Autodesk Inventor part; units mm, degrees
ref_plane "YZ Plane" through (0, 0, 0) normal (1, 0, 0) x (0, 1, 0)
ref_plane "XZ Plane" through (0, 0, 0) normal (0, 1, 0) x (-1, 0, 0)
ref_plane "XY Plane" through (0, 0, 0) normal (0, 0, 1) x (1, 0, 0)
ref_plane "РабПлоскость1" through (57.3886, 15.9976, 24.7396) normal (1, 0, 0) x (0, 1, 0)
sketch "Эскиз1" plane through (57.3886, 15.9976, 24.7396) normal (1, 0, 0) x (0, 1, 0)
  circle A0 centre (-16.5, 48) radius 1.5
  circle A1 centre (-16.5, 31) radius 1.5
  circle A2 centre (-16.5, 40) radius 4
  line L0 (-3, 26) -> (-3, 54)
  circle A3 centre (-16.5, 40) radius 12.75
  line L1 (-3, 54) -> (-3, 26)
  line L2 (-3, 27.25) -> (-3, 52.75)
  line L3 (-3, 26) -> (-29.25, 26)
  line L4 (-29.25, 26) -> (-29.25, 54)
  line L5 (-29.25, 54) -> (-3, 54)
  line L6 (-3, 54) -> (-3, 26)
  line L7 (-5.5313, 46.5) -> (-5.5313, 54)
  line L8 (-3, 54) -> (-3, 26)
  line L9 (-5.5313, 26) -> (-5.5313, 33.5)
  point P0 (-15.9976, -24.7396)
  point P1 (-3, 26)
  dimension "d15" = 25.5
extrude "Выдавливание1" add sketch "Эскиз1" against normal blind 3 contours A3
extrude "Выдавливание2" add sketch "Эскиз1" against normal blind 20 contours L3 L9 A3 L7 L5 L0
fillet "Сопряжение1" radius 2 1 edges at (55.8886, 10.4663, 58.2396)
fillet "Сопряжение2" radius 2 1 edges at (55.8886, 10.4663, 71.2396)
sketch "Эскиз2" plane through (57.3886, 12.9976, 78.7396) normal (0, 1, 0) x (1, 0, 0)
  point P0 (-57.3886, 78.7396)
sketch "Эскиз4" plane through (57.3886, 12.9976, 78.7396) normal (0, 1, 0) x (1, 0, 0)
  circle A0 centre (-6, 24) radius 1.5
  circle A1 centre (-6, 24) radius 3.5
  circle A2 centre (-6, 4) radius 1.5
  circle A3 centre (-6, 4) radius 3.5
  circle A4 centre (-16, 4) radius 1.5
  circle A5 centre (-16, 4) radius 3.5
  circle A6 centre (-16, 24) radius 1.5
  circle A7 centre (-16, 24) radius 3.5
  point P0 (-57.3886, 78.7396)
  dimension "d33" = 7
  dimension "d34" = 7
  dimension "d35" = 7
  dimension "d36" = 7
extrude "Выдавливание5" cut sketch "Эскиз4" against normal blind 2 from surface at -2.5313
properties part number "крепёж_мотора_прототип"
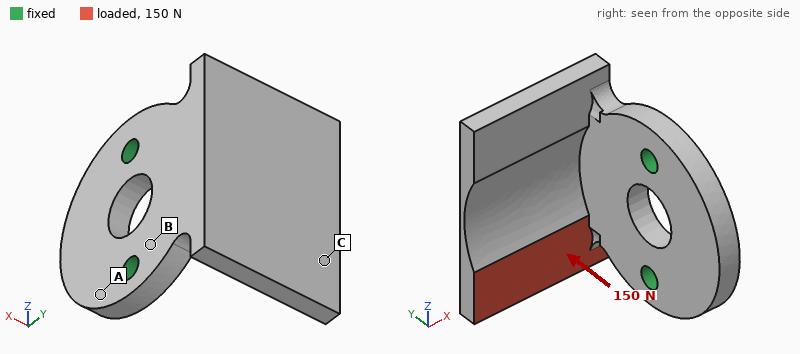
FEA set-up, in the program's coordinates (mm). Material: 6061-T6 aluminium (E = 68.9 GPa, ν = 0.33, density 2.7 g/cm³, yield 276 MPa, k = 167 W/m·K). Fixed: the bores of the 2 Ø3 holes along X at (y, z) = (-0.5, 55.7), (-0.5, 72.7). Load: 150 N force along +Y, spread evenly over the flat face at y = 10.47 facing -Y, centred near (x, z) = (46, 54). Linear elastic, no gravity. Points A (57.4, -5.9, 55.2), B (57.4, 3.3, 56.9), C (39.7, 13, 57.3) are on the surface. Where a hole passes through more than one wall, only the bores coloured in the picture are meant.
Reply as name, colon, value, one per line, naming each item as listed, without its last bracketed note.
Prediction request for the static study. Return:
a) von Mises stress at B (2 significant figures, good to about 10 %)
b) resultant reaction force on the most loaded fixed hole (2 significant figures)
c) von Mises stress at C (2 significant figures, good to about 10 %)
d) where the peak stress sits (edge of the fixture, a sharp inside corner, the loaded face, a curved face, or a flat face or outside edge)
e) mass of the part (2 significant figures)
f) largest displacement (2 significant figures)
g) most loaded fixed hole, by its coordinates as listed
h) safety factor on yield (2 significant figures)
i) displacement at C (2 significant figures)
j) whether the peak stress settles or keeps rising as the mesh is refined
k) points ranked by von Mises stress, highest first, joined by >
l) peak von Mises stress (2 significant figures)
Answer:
von Mises stress at B: 50 MPa
resultant reaction force on the most loaded fixed hole: 160 N
von Mises stress at C: 24 MPa
where the peak stress sits: a curved face
mass of the part: 6.7 g
largest displacement: 0.28 mm
most loaded fixed hole, by its coordinates as listed: (-0.5, 55.7)
safety factor on yield: 1.3
displacement at C: 0.21 mm
whether the peak stress settles or keeps rising as the mesh is refined: settles
points ranked by von Mises stress, highest first, joined by >: B > C > A
peak von Mises stress: 220 MPa
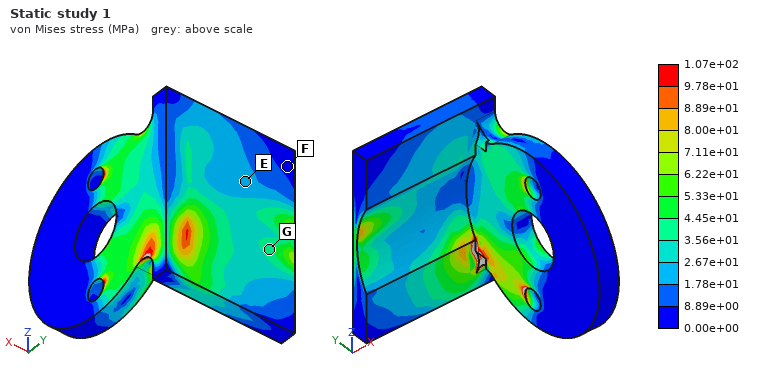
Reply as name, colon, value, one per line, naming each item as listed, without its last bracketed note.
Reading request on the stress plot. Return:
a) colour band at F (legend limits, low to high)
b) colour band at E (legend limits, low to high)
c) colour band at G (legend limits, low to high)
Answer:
colour band at F: 0.00e+00 to 8.89e+00 MPa
colour band at E: 1.78e+01 to 2.67e+01 MPa
colour band at G: 3.56e+01 to 4.45e+01 MPa
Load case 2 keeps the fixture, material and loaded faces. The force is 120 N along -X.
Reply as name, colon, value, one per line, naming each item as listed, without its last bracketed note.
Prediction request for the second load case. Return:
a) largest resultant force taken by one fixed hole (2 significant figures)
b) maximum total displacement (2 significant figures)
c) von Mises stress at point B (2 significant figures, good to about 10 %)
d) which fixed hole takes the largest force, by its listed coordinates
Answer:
largest resultant force taken by one fixed hole: 130 N
maximum total displacement: 66 µm
von Mises stress at point B: 50 MPa
which fixed hole takes the largest force, by its listed coordinates: (-0.5, 55.7)
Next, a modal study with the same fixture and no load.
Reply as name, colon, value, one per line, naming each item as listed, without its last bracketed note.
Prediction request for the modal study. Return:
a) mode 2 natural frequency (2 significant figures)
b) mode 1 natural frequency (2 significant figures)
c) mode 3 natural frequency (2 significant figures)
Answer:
mode 2 natural frequency: 5100 Hz
mode 1 natural frequency: 3200 Hz
mode 3 natural frequency: 7600 Hz
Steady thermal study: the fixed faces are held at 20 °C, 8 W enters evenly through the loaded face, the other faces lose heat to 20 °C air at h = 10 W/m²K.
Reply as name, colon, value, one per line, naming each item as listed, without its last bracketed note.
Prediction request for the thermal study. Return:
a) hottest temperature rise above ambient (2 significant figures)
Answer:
hottest temperature rise above ambient: 26 K
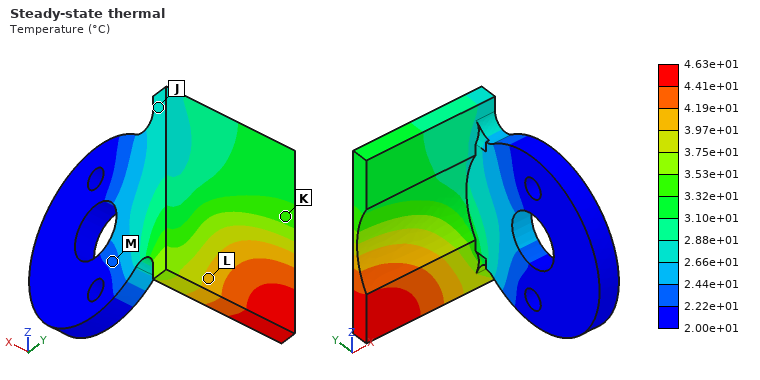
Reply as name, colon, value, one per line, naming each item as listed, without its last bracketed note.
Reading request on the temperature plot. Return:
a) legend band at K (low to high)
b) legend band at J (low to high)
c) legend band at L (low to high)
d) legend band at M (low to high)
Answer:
legend band at K: 3.32e+01 to 3.53e+01 °C
legend band at J: 2.66e+01 to 2.88e+01 °C
legend band at L: 3.97e+01 to 4.19e+01 °C
legend band at M: 2.22e+01 to 2.44e+01 °C
